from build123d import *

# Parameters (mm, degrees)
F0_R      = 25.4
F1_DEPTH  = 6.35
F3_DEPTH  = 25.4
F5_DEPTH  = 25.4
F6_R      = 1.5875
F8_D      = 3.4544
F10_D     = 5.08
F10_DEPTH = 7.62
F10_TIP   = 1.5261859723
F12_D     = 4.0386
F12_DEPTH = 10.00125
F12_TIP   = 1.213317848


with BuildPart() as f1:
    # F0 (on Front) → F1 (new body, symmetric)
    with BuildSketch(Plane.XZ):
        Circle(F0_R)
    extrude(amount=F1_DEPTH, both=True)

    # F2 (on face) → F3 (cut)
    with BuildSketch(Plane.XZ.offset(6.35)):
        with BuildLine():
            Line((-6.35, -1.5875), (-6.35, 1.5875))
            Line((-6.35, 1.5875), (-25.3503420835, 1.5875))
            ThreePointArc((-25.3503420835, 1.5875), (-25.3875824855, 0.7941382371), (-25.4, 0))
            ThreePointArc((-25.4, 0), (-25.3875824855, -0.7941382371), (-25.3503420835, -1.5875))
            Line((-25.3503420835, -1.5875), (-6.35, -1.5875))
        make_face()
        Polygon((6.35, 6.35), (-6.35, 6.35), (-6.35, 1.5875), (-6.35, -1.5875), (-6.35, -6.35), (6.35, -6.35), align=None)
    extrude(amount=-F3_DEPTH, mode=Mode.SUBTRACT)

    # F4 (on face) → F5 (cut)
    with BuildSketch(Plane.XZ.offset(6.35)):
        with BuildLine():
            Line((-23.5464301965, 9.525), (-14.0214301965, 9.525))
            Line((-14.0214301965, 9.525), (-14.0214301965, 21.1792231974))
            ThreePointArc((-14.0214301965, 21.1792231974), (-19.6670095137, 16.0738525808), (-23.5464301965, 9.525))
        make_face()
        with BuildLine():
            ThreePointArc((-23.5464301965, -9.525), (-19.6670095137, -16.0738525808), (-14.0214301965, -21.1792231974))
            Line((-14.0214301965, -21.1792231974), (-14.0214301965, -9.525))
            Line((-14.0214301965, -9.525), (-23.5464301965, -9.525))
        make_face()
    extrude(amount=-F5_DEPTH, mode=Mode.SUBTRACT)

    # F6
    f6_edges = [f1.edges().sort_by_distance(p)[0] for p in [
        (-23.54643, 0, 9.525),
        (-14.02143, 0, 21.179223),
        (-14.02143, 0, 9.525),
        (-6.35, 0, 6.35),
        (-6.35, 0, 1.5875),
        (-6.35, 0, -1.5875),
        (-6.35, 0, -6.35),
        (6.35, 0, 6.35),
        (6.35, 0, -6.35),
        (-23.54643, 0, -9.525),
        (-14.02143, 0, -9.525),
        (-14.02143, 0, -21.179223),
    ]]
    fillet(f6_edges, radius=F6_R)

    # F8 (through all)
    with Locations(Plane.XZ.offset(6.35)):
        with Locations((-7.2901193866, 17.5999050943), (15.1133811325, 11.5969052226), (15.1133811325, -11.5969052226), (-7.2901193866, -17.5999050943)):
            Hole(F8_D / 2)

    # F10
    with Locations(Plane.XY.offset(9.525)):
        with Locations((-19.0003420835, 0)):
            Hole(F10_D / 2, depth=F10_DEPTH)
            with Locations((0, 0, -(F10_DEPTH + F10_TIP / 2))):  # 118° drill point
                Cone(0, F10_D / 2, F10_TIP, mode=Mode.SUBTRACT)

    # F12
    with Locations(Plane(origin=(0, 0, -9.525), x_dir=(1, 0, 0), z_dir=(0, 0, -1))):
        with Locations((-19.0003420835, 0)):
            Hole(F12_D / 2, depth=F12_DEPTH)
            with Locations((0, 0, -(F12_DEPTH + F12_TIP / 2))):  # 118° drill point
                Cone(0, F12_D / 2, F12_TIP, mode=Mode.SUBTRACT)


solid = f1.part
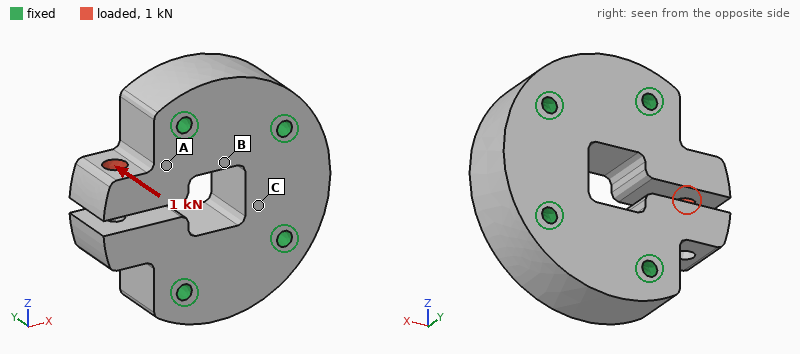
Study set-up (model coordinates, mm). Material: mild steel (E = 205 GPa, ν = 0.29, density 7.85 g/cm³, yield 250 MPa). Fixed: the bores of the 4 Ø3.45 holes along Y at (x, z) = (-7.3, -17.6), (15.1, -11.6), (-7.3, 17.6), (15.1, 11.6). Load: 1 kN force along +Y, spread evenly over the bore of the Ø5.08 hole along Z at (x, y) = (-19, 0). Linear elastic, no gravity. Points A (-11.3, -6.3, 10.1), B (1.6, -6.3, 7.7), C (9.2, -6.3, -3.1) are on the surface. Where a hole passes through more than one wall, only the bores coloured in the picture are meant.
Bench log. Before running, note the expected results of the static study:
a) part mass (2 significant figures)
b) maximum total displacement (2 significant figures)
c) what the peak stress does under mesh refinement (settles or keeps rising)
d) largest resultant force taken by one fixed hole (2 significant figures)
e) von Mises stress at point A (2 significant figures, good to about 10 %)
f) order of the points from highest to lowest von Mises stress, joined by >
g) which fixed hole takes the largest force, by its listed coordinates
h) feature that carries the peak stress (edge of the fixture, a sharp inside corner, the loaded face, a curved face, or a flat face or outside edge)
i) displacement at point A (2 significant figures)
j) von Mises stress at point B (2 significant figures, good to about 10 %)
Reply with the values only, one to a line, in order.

160 g
12 µm
keeps rising
1.2 kN
47 MPa
A > B > C
(-7.3, 17.6)
edge of the fixture
2.9 µm
14 MPa
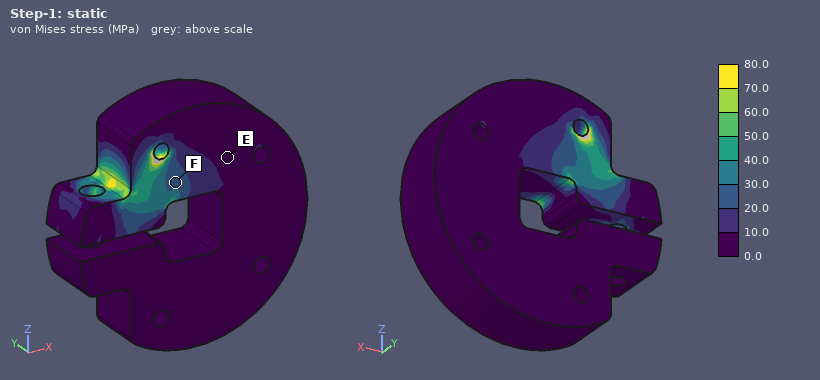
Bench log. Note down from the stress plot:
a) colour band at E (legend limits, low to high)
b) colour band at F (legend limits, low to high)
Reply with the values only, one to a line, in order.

0.0 to 10.0 MPa
20.0 to 30.0 MPa
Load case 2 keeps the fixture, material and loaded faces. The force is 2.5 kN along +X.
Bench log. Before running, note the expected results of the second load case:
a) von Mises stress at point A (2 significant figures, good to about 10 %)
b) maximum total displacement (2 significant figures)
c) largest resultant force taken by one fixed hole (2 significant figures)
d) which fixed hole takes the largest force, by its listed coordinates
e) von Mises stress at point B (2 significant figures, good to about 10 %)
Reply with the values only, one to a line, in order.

27 MPa
11 µm
1.6 kN
(-7.3, 17.6)
26 MPa
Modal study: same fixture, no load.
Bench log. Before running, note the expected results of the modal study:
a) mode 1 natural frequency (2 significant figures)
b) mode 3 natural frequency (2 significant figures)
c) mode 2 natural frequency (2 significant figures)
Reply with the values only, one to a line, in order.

18 kHz
19 kHz
18 kHz
